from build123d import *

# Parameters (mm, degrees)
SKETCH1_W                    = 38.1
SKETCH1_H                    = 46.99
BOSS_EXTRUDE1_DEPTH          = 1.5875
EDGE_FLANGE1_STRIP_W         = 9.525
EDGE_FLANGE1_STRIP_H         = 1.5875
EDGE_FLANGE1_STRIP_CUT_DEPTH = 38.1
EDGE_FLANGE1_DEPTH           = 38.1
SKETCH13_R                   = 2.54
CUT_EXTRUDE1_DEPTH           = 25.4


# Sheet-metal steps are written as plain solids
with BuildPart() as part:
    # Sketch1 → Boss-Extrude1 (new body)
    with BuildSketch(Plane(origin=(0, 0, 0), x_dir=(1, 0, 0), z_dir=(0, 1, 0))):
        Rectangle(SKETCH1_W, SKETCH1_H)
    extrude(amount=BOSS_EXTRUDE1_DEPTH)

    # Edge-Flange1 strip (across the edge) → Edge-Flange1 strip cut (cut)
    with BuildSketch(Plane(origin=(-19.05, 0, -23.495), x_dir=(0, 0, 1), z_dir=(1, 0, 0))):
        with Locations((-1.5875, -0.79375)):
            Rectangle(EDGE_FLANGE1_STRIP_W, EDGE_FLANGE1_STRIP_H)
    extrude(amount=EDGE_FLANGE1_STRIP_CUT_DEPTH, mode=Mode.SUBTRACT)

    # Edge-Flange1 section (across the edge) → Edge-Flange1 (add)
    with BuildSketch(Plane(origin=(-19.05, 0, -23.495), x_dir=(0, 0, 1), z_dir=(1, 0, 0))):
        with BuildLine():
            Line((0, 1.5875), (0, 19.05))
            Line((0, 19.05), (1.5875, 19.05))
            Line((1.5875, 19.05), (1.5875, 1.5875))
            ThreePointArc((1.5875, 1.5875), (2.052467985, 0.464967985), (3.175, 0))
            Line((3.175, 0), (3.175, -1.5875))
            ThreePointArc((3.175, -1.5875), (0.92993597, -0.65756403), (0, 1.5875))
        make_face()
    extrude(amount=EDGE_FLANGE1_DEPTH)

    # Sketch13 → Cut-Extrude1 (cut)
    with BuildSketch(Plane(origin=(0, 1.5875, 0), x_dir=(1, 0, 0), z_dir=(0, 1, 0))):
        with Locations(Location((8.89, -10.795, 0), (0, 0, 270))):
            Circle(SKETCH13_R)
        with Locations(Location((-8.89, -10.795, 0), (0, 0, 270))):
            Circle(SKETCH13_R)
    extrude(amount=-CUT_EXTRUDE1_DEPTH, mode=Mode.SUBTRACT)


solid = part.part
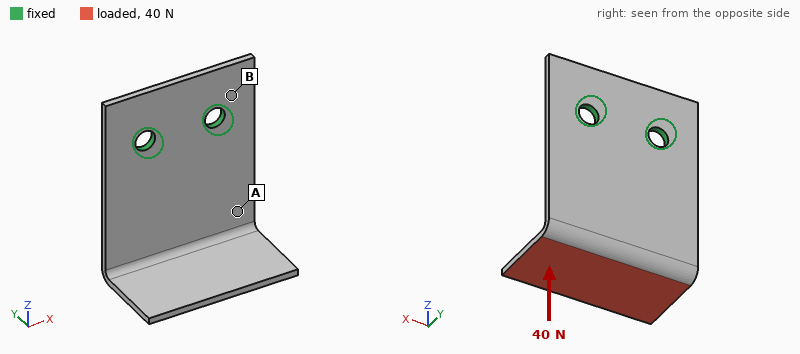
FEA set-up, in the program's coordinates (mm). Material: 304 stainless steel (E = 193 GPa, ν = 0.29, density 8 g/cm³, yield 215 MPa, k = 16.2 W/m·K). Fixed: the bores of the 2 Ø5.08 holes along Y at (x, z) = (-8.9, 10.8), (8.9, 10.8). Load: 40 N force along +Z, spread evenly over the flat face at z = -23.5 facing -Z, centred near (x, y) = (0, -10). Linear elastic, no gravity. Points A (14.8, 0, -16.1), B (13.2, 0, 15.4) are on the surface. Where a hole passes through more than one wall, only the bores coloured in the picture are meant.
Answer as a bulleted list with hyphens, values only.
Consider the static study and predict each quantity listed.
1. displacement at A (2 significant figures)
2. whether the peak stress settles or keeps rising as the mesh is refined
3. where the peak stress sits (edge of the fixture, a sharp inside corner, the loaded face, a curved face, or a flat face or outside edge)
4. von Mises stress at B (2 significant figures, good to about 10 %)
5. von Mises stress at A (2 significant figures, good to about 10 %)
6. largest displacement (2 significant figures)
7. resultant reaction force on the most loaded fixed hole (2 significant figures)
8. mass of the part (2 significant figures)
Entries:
- 0.057 mm
- keeps rising
- edge of the fixture
- 3.6 MPa
- 27 MPa
- 0.16 mm
- 20 N
- 31 g
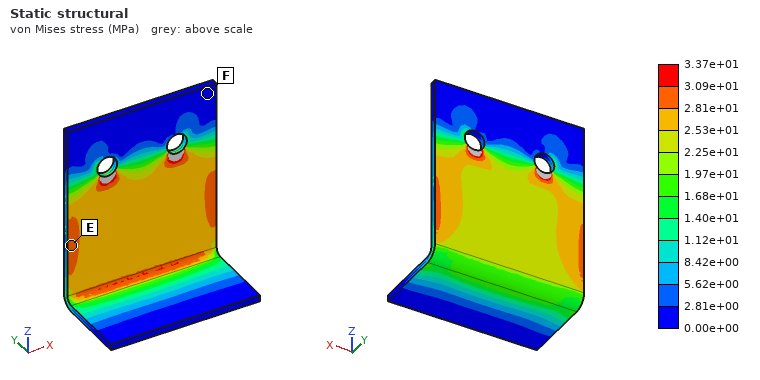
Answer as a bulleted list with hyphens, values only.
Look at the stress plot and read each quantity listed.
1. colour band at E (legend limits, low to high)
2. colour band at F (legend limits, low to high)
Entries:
- 2.81e+01 to 3.09e+01 MPa
- 0.00e+00 to 2.81e+00 MPa
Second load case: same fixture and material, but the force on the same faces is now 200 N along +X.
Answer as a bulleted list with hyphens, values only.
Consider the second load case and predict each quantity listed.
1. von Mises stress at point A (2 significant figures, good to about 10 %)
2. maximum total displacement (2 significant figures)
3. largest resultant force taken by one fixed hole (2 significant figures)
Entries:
- 92 MPa
- 0.34 mm
- 340 N
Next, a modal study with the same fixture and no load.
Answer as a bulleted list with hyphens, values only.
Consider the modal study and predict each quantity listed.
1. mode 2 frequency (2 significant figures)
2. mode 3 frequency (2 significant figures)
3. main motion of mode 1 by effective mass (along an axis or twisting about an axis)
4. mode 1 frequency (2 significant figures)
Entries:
- 1200 Hz
- 2100 Hz
- along Y
- 610 Hz
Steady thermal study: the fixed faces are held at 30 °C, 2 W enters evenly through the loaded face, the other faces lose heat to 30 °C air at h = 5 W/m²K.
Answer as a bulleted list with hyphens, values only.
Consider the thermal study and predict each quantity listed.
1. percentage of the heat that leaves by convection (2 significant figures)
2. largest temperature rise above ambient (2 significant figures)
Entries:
- 31 %
- 69 K
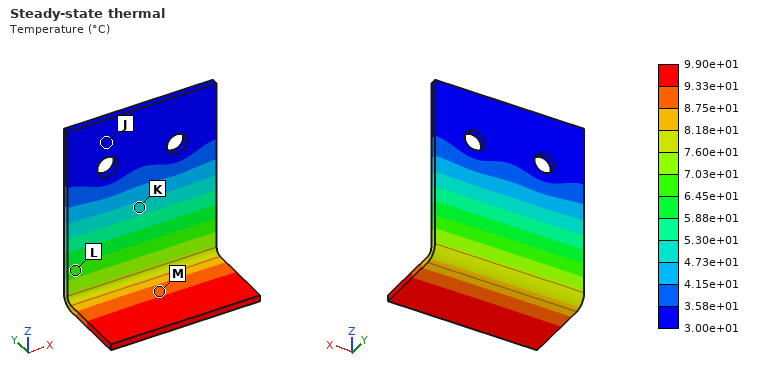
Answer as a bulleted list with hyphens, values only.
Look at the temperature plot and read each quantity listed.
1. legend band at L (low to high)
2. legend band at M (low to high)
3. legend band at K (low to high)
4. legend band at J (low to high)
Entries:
- 6.45e+01 to 7.03e+01 °C
- 8.75e+01 to 9.33e+01 °C
- 4.73e+01 to 5.30e+01 °C
- 3.00e+01 to 3.58e+01 °C
